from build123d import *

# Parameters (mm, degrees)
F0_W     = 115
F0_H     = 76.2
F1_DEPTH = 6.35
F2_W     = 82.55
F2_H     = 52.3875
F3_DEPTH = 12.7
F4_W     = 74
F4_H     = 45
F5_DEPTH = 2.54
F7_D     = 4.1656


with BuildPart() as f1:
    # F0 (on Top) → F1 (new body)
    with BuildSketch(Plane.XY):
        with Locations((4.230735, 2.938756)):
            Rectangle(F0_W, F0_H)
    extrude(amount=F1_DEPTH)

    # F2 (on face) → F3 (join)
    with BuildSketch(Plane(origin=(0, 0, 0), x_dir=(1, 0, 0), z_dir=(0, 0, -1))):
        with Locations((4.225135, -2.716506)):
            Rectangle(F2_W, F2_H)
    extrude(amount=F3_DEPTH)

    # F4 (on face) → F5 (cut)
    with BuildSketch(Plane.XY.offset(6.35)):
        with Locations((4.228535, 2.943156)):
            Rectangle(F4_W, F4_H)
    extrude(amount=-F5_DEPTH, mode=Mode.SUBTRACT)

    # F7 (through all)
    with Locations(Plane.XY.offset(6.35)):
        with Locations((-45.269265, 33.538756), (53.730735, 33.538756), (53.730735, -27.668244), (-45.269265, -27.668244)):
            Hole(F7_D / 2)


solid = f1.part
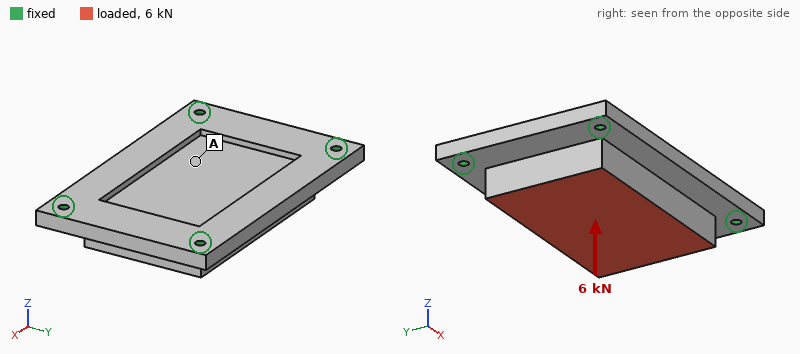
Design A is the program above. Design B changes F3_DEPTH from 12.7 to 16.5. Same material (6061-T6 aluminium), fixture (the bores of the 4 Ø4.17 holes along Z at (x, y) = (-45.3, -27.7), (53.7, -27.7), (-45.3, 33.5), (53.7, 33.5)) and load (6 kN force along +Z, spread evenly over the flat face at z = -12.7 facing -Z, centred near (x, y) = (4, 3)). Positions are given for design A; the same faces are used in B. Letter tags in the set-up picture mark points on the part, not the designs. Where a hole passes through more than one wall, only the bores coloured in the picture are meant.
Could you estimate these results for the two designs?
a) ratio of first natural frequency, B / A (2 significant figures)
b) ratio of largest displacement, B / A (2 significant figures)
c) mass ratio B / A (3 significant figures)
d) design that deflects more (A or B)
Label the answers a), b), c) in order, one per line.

a) 1.0
b) 0.81
c) 1.16
d) A
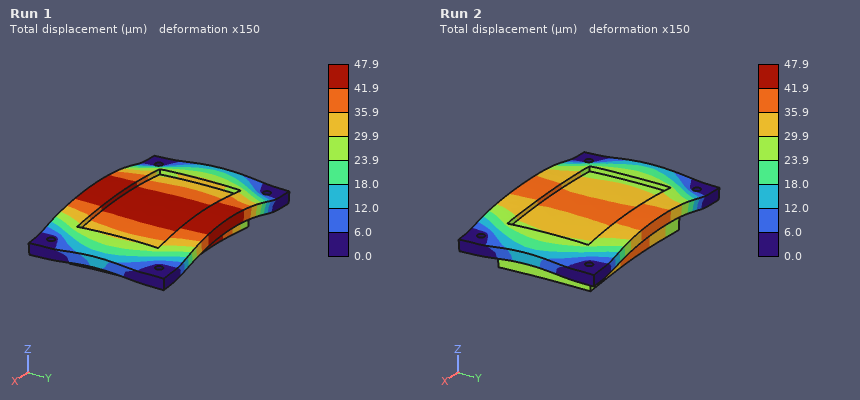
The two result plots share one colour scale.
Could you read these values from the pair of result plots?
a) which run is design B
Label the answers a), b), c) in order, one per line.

a) Run 2
